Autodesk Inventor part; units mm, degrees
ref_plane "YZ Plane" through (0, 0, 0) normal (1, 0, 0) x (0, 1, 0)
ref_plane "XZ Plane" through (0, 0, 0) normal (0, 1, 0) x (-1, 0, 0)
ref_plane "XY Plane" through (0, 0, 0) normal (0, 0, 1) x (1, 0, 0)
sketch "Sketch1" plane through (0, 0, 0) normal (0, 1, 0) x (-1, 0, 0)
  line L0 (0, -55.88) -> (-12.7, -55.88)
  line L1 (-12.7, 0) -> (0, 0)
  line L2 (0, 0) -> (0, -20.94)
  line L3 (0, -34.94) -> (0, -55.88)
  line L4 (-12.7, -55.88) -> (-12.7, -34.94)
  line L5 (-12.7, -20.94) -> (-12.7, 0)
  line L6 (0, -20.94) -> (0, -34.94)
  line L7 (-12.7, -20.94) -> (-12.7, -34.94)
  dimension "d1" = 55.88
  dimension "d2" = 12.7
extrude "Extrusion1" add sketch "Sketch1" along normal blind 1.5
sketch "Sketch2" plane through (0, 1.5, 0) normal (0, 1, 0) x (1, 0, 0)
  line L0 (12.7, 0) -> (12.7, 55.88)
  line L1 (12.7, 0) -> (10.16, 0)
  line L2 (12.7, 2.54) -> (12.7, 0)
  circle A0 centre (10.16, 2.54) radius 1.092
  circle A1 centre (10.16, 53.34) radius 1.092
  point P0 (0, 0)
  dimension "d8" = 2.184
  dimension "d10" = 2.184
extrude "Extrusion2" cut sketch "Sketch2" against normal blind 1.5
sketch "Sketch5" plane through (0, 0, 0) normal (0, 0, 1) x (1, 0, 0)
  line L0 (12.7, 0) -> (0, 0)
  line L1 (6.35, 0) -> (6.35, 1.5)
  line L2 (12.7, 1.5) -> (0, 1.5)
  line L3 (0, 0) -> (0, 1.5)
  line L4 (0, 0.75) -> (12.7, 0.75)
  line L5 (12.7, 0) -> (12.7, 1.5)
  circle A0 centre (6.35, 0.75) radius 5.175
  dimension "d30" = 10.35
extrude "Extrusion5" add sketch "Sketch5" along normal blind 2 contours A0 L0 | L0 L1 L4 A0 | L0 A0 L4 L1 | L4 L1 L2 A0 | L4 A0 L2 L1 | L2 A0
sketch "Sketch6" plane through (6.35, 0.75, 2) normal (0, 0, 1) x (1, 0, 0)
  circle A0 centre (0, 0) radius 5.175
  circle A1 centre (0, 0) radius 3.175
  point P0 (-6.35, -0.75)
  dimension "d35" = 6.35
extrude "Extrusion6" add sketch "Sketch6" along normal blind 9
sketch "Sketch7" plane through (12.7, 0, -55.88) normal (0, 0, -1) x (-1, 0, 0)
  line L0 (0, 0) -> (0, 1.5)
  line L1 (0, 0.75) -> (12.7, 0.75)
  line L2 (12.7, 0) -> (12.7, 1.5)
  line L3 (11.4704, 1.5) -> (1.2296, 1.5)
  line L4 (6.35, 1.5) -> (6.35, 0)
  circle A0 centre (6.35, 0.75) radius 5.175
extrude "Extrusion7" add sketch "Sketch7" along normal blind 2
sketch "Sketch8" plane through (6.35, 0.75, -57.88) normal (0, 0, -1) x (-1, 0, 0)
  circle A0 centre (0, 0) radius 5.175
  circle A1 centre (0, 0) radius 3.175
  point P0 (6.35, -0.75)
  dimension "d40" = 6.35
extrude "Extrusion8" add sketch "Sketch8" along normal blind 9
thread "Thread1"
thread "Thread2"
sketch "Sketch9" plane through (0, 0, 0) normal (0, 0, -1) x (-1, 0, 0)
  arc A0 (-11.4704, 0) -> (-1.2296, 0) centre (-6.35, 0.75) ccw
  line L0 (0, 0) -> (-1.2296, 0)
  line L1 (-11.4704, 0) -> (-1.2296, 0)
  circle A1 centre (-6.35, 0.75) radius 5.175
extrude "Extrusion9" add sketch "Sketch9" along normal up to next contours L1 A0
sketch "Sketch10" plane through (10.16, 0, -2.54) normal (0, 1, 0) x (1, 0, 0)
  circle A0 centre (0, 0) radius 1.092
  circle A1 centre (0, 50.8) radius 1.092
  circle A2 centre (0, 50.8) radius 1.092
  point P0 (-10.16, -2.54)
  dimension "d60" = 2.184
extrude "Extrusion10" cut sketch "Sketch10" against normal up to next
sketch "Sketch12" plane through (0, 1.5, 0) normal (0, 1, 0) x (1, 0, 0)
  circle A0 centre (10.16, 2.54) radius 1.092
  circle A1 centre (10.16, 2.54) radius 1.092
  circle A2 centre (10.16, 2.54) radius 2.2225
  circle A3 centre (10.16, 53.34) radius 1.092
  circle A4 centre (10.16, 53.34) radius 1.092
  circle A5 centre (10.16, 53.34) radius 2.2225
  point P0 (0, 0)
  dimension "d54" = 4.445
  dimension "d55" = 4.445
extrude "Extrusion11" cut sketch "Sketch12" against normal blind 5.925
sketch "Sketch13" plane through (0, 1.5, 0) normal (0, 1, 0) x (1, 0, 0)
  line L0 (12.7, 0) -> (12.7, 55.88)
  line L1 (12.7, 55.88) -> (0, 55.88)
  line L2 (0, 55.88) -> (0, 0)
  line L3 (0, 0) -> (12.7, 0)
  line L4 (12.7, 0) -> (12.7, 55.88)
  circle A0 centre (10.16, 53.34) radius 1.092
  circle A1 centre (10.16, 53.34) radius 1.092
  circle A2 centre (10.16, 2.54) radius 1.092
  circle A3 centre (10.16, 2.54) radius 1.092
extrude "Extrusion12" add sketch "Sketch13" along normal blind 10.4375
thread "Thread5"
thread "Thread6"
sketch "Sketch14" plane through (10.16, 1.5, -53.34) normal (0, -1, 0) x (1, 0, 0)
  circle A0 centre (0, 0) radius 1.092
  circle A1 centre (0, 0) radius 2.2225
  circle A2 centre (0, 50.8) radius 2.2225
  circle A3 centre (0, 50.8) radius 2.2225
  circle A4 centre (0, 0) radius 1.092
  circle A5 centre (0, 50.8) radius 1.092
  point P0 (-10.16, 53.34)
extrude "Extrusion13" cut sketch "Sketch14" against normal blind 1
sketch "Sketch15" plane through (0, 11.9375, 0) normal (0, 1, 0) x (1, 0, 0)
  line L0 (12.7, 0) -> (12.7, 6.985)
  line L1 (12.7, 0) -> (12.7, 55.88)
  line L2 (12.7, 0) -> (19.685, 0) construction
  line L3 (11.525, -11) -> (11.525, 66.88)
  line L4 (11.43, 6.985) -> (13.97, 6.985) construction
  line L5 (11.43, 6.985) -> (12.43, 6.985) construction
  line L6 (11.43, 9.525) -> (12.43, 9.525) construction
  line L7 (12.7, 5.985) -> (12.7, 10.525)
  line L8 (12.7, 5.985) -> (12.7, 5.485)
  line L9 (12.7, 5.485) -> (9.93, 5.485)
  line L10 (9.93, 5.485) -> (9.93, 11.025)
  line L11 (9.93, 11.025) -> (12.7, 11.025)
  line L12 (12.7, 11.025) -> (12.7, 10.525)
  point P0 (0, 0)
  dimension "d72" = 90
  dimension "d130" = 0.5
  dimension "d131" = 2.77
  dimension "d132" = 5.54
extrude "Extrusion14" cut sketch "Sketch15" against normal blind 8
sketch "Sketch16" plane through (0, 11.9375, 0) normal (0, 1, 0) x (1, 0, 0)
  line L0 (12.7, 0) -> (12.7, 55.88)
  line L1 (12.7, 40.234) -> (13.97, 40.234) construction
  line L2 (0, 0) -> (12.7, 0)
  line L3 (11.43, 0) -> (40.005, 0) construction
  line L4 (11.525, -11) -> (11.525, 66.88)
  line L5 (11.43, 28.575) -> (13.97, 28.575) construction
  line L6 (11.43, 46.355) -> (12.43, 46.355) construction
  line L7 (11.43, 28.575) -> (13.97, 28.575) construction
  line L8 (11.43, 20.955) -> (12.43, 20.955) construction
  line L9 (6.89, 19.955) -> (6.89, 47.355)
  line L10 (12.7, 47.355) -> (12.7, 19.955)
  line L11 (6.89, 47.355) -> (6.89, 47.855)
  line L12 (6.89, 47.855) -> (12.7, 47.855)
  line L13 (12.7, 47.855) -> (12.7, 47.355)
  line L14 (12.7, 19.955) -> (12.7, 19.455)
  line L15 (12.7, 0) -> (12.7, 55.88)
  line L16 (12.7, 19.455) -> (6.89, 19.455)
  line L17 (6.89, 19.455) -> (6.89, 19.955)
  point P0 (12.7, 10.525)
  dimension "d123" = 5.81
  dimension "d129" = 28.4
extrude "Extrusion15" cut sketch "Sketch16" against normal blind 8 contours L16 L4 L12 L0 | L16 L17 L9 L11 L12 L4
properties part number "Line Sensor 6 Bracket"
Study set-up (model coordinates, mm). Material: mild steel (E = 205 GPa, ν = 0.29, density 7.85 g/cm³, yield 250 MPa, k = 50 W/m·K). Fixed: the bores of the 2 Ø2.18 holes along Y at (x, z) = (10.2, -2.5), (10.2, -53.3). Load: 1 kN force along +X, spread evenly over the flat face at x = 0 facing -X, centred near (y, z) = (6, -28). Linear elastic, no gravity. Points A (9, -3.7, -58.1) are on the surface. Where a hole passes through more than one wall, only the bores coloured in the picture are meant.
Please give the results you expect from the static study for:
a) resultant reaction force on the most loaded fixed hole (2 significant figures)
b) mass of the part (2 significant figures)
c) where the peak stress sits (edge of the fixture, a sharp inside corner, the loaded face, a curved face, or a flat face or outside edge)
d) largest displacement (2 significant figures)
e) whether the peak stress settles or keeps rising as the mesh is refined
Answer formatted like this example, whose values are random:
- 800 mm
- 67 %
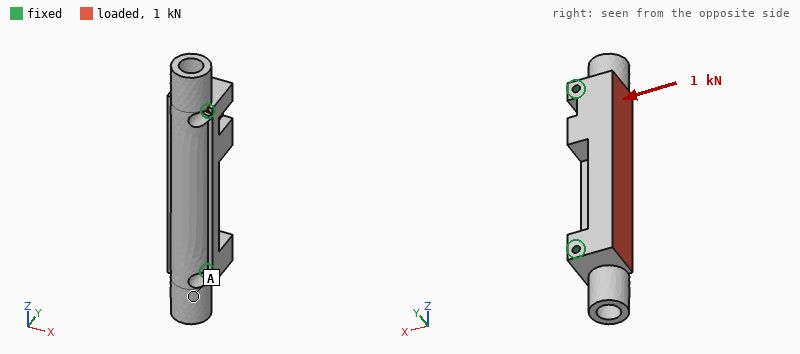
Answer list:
- 650 N
- 79 g
- edge of the fixture
- 3.3 µm
- keeps rising
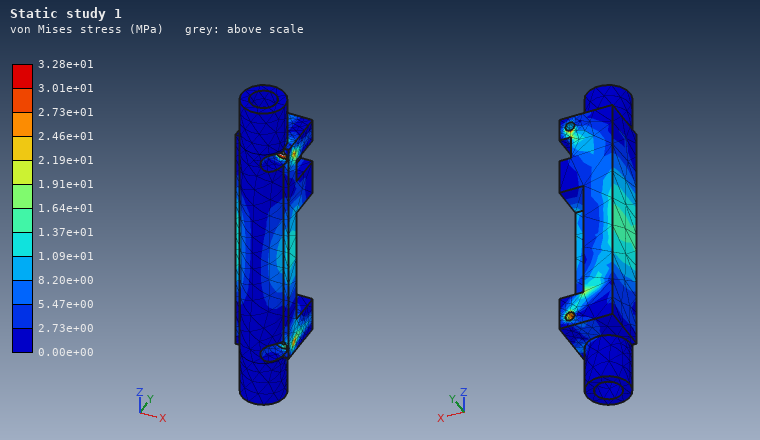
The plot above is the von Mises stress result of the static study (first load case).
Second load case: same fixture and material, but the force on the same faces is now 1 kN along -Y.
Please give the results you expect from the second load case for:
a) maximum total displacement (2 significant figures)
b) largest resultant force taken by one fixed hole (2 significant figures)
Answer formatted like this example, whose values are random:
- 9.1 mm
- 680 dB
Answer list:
- 4.9 µm
- 530 N
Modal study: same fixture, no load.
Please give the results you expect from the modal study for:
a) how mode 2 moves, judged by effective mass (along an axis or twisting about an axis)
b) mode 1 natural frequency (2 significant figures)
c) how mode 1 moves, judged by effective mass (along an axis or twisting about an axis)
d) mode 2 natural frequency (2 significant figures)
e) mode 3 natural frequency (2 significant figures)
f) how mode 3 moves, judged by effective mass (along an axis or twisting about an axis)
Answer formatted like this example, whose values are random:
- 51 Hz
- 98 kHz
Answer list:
- along Y
- 12 kHz
- along X
- 14 kHz
- 18 kHz
- twisting about Z
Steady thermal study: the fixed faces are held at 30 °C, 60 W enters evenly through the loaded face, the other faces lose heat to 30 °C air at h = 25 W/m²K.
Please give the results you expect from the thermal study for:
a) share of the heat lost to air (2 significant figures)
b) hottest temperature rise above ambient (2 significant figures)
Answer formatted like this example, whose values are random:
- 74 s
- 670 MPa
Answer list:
- 6.1 %
- 75 K
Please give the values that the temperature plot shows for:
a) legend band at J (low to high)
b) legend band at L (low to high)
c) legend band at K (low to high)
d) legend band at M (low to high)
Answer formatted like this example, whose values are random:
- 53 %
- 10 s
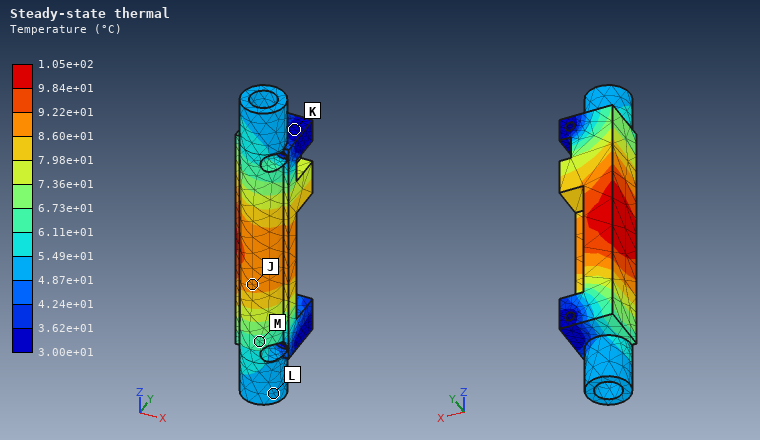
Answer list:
- 8.60e+01 to 9.22e+01 °C
- 4.87e+01 to 5.49e+01 °C
- 3.00e+01 to 3.62e+01 °C
- 6.11e+01 to 6.73e+01 °C
